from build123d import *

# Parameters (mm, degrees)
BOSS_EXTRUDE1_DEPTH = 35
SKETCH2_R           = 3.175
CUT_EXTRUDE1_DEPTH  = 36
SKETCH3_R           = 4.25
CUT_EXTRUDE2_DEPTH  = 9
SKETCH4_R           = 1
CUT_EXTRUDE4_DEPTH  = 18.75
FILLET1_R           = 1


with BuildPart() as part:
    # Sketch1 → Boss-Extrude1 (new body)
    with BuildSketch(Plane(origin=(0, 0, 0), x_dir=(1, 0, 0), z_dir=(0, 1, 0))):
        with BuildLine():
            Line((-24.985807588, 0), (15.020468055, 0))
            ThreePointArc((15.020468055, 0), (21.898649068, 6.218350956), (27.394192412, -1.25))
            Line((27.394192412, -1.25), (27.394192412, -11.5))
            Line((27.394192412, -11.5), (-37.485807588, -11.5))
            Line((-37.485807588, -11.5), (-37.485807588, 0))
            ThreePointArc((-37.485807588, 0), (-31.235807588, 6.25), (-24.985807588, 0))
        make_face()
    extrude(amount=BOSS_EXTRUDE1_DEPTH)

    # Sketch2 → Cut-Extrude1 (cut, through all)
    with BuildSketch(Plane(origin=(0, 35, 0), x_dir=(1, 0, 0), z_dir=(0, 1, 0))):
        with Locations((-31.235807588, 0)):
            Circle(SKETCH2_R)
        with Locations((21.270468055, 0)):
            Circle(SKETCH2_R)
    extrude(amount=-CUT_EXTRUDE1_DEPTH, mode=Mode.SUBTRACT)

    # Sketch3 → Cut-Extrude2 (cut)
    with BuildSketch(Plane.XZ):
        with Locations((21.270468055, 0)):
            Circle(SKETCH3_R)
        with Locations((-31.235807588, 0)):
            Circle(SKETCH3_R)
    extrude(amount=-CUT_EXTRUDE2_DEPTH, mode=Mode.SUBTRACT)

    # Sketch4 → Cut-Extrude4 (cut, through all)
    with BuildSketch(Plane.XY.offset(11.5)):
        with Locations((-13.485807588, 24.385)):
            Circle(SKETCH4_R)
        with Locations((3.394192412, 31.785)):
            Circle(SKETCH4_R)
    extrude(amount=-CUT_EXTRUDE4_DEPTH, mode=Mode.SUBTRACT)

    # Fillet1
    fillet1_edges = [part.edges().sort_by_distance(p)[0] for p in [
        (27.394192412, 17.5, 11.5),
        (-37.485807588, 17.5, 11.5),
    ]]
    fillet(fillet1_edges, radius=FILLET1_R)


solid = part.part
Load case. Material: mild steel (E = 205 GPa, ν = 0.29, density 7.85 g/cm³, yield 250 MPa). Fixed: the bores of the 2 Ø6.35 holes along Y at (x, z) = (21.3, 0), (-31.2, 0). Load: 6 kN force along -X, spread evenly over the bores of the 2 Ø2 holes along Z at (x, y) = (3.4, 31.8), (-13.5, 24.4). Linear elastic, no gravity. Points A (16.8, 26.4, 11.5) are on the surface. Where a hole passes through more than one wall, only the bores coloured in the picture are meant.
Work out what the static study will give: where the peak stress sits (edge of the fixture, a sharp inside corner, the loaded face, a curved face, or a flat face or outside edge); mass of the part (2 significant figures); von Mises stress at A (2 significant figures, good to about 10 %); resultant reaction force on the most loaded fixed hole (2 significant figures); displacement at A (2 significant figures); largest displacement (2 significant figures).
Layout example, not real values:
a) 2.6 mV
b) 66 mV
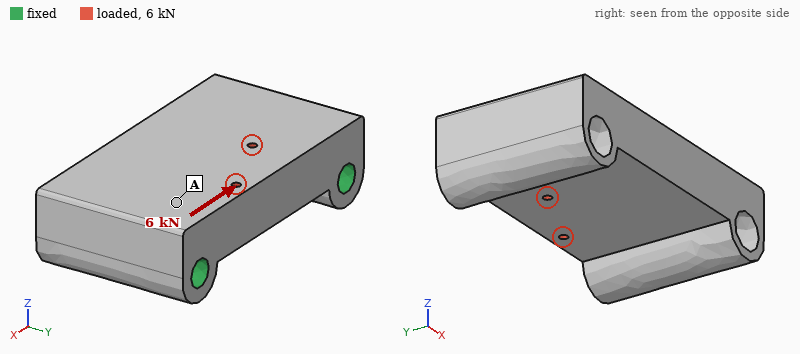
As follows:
a) the loaded face
b) 220 g
c) 7.2 MPa
d) 3.1 kN
e) 0.92 µm
f) 2.3 µm
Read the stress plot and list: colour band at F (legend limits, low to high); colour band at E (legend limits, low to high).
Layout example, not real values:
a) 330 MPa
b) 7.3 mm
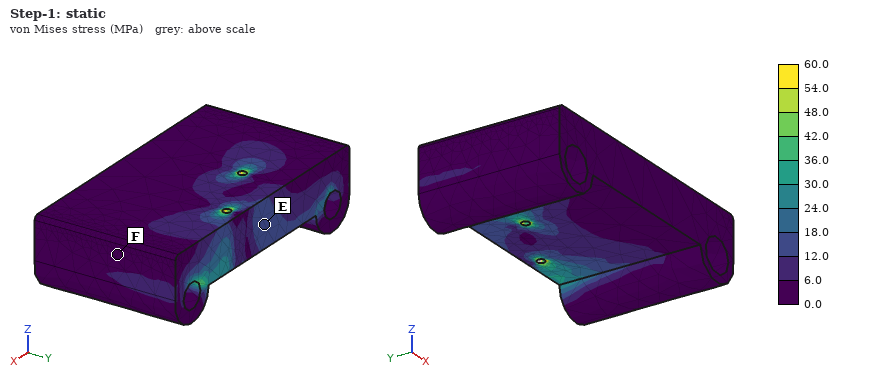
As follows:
a) 0.0 to 6.0 MPa
b) 12.0 to 18.0 MPa
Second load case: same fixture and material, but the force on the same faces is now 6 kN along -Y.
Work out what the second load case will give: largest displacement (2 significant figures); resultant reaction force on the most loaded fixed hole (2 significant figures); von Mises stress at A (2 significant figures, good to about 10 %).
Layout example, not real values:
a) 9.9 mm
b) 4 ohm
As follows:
a) 4.0 µm
b) 3.0 kN
c) 9.6 MPa
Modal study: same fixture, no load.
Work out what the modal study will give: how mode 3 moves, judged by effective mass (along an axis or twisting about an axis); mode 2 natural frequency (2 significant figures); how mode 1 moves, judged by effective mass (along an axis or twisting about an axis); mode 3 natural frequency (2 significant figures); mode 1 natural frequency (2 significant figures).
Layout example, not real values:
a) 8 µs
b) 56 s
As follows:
a) along Y
b) 21 kHz
c) along Z
d) 24 kHz
e) 16 kHz
